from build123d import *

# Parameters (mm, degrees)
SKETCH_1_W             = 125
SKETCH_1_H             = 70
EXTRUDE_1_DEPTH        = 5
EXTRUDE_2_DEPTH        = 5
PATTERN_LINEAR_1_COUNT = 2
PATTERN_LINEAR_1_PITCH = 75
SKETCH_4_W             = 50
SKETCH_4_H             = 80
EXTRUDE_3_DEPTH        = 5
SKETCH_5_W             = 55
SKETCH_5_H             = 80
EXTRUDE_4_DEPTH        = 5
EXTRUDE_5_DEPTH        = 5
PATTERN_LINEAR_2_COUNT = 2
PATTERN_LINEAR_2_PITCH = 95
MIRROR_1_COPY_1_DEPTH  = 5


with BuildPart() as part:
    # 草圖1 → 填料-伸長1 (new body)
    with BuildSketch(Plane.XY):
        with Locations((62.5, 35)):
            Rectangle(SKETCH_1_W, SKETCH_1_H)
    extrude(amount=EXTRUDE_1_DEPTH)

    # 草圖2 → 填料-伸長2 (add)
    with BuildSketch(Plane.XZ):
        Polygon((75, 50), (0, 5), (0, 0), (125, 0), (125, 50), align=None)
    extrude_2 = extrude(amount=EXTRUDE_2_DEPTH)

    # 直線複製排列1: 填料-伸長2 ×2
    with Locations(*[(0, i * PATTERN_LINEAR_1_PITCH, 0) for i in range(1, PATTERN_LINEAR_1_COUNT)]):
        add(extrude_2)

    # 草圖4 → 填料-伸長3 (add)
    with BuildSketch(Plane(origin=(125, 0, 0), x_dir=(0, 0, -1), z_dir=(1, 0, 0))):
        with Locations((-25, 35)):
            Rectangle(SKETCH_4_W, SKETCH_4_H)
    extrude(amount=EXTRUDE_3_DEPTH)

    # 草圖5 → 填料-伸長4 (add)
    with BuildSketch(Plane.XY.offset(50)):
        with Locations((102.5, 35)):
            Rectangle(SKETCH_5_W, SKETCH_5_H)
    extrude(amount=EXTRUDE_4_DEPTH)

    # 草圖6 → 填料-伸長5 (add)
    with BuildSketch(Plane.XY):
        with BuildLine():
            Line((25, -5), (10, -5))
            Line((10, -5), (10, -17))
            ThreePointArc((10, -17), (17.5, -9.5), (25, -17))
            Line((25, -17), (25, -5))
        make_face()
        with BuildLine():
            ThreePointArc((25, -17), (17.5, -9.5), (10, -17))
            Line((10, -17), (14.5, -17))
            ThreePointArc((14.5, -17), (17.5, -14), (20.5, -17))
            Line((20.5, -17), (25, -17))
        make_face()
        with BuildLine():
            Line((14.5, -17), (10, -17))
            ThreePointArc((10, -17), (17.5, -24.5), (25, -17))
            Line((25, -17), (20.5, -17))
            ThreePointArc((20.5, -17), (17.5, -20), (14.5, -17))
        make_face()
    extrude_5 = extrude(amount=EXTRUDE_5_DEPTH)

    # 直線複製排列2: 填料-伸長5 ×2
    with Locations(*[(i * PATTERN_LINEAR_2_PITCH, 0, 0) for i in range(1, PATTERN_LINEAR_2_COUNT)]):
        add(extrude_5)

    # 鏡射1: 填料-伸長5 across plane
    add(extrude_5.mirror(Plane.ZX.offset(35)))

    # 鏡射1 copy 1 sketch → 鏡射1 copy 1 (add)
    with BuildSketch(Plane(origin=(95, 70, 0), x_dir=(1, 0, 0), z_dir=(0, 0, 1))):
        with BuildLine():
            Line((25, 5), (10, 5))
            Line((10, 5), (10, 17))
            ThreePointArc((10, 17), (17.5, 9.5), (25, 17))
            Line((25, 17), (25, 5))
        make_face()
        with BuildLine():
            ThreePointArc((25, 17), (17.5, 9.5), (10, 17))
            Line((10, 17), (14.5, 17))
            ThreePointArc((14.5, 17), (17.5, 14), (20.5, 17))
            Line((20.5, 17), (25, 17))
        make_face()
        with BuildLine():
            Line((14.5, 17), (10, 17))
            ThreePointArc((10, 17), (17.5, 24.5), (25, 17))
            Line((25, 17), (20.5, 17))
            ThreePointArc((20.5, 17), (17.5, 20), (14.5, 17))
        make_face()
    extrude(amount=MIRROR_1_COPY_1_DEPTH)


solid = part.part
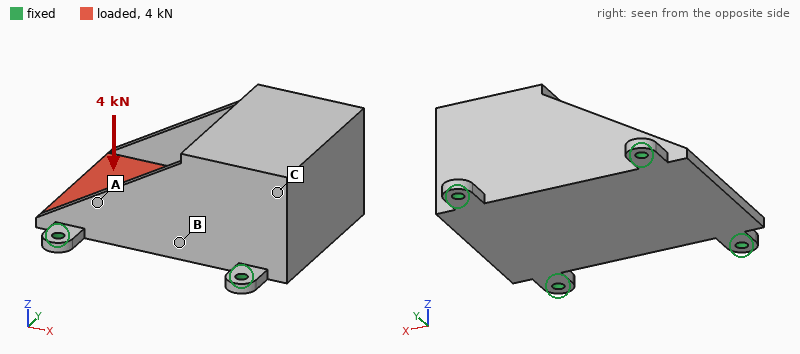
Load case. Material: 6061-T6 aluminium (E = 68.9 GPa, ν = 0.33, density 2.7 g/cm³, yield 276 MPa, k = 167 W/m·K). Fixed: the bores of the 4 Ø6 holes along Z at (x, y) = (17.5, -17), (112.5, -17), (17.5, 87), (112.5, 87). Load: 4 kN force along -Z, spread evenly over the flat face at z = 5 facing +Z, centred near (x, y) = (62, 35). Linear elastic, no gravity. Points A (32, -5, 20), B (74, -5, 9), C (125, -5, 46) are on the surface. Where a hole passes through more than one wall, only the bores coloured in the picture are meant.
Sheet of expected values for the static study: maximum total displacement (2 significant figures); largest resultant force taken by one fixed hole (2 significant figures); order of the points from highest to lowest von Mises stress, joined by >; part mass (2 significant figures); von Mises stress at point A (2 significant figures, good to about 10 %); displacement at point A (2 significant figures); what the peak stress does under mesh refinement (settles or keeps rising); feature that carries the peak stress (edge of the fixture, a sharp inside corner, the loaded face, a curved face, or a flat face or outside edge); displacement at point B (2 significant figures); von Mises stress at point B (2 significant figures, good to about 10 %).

0.29 mm
1.1 kN
A > B > C
370 g
36 MPa
0.11 mm
keeps rising
edge of the fixture
0.051 mm
24 MPa
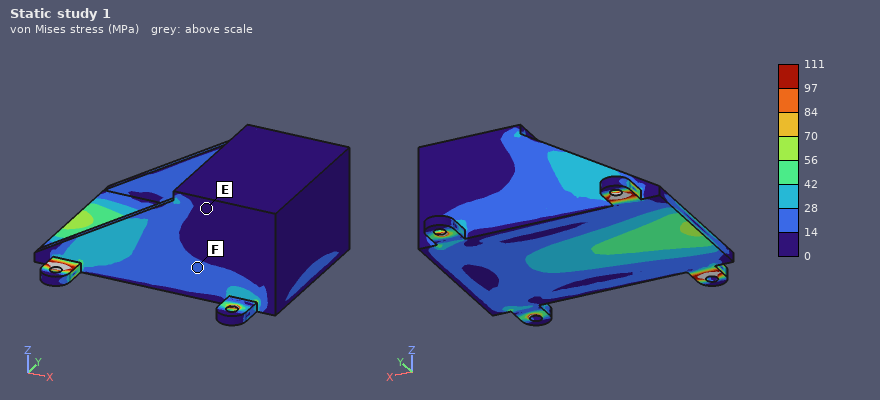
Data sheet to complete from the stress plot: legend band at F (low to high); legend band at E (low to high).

14 to 28 MPa
0 to 14 MPa
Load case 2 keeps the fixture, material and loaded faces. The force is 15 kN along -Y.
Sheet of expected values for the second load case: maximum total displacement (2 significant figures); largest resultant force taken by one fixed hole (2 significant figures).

32 µm
3.9 kN
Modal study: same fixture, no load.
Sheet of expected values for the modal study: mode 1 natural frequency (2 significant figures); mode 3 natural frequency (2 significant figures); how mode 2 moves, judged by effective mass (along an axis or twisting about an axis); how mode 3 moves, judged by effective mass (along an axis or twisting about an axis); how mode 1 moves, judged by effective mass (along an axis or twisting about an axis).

2000 Hz
2500 Hz
along Y
along Z
along Z
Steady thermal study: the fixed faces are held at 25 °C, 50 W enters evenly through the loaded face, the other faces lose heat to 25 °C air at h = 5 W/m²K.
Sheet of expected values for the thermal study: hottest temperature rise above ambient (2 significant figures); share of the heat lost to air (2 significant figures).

20 K
6.9 %
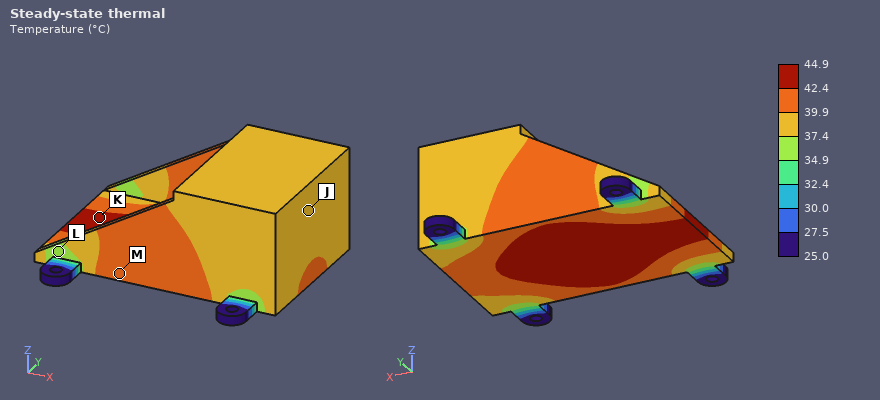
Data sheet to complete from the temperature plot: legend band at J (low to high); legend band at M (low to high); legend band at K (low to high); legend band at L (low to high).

37.4 to 39.9 °C
39.9 to 42.4 °C
42.4 to 44.9 °C
34.9 to 37.4 °C
